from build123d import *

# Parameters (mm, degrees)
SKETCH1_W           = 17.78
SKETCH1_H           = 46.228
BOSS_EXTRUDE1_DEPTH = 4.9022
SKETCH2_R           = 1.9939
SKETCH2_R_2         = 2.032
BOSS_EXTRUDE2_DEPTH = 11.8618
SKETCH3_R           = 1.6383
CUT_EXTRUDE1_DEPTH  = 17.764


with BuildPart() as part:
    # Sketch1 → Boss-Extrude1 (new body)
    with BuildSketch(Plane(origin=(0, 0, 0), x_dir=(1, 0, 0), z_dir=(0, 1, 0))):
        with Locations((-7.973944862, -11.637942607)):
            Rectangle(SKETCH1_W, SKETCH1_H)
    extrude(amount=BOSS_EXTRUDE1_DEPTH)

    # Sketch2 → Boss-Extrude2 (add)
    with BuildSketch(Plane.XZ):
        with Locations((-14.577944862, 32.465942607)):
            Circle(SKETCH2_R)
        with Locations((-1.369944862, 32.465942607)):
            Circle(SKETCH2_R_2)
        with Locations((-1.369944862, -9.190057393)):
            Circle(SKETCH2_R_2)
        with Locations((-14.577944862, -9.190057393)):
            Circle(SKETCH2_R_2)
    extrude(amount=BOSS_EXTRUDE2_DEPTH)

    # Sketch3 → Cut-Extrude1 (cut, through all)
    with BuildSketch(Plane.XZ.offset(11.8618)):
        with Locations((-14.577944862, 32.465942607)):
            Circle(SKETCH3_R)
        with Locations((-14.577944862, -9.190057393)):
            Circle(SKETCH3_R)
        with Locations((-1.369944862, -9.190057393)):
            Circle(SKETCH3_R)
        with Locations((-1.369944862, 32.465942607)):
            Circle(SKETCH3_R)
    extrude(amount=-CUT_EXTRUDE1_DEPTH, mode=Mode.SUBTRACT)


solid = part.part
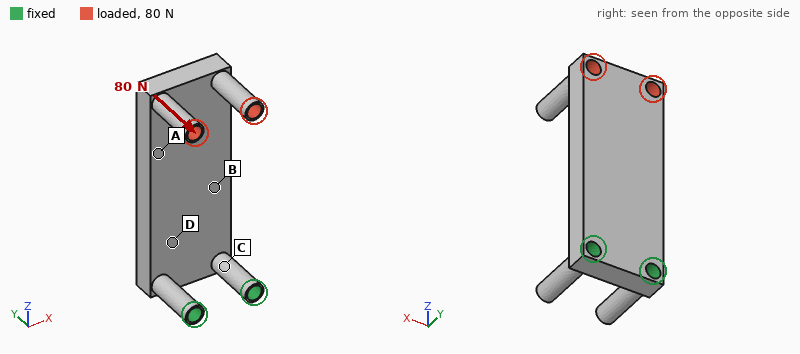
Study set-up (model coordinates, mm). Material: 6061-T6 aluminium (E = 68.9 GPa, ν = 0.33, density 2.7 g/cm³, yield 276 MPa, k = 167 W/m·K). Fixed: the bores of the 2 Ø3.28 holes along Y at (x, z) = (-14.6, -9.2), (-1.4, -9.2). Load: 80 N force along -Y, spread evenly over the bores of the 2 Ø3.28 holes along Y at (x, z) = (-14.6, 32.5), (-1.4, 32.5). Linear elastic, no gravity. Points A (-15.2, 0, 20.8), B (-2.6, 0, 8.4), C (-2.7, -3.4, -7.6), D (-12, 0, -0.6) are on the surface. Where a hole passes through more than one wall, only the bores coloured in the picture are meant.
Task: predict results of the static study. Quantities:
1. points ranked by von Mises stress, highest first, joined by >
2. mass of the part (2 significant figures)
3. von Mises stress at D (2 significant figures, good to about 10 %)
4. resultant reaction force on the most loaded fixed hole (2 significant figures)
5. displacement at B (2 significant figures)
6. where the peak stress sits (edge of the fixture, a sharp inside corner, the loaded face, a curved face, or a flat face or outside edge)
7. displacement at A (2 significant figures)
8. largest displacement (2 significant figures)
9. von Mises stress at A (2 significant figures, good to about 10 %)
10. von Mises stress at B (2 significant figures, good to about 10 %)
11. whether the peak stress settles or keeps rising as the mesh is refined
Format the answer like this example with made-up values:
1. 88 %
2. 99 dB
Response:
1. D > B > A > C
2. 11 g
3. 36 MPa
4. 40 N
5. 0.037 mm
6. edge of the fixture
7. 0.094 mm
8. 0.19 mm
9. 13 MPa
10. 27 MPa
11. keeps rising
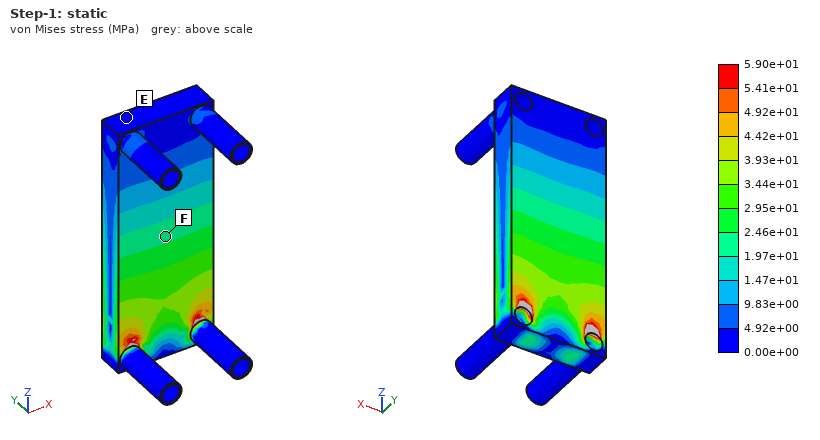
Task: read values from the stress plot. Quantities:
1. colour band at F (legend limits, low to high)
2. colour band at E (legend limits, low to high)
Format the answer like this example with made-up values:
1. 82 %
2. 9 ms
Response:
1. 1.97e+01 to 2.46e+01 MPa
2. 0.00e+00 to 4.92e+00 MPa
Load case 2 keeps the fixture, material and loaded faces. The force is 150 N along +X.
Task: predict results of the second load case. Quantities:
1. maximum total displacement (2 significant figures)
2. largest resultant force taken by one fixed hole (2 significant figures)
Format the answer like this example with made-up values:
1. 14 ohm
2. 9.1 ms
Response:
1. 0.10 mm
2. 460 N
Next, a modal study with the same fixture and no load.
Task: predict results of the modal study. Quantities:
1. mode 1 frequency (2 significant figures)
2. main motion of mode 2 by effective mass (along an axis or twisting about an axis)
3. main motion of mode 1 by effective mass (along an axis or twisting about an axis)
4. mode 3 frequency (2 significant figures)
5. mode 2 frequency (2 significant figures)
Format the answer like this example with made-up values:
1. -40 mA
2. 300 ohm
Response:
1. 2100 Hz
2. along X
3. along Y
4. 8700 Hz
5. 6900 Hz
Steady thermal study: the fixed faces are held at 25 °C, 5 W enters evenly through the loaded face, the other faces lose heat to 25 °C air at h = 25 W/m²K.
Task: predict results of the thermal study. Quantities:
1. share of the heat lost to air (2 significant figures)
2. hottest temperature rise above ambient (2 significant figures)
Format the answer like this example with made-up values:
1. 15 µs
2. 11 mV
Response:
1. 11 %
2. 29 K
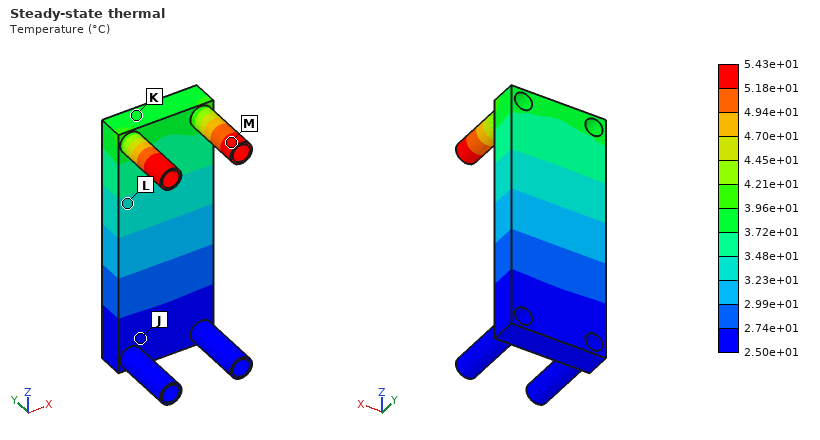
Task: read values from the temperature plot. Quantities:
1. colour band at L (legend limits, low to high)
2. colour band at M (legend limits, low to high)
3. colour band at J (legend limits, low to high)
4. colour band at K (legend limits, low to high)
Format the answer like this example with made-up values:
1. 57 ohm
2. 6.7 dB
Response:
1. 3.23e+01 to 3.48e+01 °C
2. 5.18e+01 to 5.43e+01 °C
3. 2.50e+01 to 2.74e+01 °C
4. 3.72e+01 to 3.96e+01 °C
